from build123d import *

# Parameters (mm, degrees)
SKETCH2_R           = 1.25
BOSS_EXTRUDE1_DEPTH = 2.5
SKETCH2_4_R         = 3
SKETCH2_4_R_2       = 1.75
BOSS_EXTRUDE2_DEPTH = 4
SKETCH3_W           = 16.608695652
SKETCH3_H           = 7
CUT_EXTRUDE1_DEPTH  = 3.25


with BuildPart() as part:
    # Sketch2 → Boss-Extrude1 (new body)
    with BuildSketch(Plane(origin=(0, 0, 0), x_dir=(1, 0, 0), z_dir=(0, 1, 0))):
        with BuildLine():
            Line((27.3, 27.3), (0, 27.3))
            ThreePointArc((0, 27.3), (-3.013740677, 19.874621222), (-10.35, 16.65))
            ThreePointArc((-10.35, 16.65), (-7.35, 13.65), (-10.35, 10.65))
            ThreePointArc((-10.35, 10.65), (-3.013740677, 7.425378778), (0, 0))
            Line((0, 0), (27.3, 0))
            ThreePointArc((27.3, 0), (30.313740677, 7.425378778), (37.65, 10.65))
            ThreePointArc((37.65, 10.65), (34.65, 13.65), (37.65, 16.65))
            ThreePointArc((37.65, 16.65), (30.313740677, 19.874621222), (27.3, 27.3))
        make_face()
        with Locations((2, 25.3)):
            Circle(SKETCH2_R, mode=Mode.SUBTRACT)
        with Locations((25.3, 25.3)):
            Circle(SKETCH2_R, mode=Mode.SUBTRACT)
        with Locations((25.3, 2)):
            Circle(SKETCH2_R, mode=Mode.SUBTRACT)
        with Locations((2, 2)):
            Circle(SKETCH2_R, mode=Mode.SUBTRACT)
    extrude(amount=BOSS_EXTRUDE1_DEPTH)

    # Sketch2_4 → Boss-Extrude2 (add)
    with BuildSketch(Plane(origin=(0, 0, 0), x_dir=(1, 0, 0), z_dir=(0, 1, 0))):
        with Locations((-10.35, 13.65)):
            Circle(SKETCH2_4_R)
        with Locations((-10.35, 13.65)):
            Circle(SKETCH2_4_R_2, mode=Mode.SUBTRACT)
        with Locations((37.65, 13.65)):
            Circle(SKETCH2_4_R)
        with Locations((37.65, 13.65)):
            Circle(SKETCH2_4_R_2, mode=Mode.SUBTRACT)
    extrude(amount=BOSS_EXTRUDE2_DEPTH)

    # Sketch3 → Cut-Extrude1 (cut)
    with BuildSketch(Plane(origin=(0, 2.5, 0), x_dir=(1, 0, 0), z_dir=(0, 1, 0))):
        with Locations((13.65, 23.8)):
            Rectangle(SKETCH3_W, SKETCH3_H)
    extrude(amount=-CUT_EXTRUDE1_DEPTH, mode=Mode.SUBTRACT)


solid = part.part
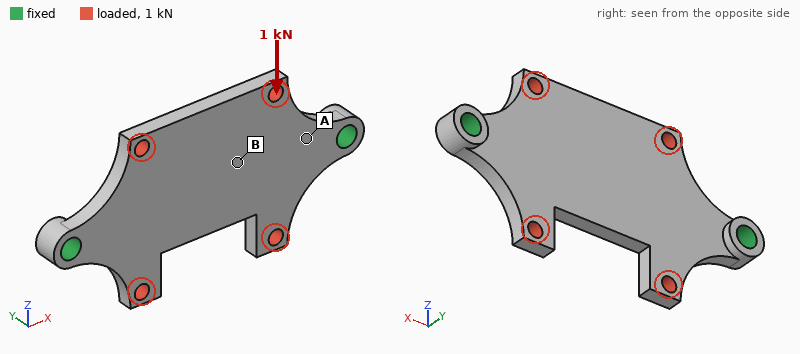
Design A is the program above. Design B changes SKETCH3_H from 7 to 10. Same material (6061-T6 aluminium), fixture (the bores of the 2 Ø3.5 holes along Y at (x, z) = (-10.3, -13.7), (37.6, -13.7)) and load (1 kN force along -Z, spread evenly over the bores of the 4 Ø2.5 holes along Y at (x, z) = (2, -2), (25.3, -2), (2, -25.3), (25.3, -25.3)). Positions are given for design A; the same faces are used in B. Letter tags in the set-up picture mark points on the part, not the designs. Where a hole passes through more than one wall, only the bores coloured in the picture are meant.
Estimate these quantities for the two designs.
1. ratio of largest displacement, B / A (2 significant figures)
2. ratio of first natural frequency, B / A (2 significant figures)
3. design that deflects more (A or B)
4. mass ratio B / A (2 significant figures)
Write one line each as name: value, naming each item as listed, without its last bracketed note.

ratio of largest displacement, B / A: 1.2
ratio of first natural frequency, B / A: 1.00
design that deflects more: B
mass ratio B / A: 0.97
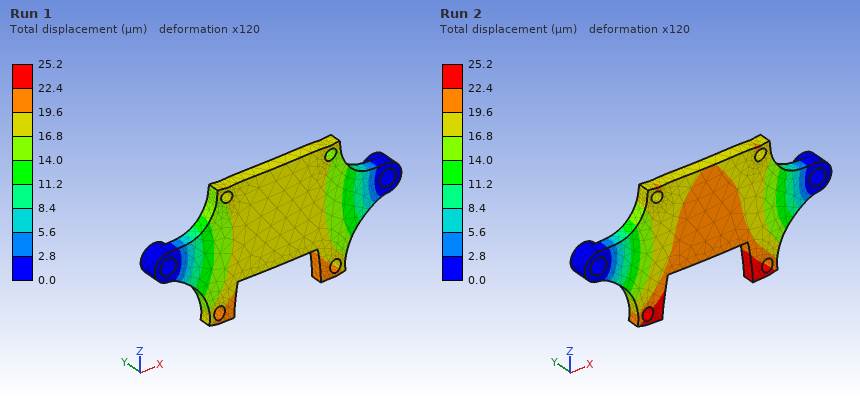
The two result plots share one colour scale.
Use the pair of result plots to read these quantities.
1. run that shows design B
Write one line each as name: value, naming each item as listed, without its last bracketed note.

run that shows design B: Run 2
